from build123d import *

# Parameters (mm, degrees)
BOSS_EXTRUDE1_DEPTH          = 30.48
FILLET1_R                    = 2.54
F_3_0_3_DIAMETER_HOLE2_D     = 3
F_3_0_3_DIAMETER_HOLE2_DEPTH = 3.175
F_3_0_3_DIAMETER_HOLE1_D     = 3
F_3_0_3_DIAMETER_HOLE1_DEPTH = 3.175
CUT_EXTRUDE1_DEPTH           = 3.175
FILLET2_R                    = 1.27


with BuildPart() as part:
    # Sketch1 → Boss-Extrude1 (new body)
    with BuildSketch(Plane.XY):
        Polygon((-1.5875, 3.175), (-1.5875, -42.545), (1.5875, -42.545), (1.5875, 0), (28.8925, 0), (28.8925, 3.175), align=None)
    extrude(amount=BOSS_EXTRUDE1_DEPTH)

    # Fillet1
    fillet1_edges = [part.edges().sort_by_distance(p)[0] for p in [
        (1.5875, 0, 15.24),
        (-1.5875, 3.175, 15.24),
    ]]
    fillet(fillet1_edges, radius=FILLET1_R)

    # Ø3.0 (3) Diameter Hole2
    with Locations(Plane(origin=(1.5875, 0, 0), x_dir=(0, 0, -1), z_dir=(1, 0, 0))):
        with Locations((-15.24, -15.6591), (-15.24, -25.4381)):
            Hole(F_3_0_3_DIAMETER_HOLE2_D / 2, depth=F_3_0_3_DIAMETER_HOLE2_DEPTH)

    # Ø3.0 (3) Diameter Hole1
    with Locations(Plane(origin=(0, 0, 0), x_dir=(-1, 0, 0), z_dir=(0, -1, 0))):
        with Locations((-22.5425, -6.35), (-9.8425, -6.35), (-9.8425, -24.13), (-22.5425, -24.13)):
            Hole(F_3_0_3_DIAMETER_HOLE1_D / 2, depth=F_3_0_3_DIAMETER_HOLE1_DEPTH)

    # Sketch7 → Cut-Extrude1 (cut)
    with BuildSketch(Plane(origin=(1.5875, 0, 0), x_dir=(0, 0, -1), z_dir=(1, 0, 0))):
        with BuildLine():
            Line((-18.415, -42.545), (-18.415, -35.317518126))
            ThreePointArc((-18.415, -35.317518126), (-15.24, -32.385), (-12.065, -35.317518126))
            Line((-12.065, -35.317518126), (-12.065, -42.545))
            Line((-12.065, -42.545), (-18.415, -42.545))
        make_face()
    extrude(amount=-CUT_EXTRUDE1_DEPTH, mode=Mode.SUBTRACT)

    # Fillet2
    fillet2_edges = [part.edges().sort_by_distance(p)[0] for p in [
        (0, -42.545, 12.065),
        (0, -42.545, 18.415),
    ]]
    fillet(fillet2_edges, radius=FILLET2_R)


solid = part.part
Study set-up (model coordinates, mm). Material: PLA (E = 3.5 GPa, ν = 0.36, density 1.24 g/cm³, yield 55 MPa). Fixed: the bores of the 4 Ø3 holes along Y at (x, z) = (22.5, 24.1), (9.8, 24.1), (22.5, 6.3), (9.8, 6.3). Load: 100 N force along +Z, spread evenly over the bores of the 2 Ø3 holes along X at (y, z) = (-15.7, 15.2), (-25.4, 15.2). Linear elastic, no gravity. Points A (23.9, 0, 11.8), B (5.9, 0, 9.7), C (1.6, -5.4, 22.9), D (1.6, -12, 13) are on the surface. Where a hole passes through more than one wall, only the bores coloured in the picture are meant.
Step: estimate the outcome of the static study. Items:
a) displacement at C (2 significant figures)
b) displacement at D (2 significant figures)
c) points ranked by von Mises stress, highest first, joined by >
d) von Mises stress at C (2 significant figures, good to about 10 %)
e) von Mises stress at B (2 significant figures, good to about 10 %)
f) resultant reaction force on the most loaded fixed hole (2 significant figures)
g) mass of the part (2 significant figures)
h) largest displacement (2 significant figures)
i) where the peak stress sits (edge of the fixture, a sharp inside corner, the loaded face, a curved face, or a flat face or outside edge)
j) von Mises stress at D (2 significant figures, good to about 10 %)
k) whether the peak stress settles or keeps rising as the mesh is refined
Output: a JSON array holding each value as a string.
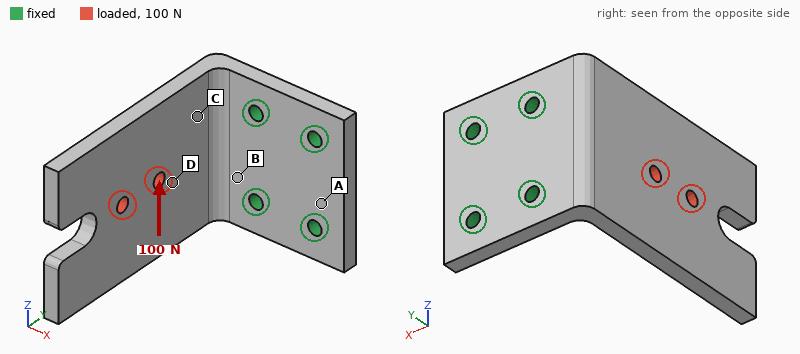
["0.14 mm", "0.20 mm", "B > C > D > A", "8.5 MPa", "12 MPa", "130 N", "8.4 g", "0.67 mm", "edge of the fixture", "4.3 MPa", "keeps rising"]
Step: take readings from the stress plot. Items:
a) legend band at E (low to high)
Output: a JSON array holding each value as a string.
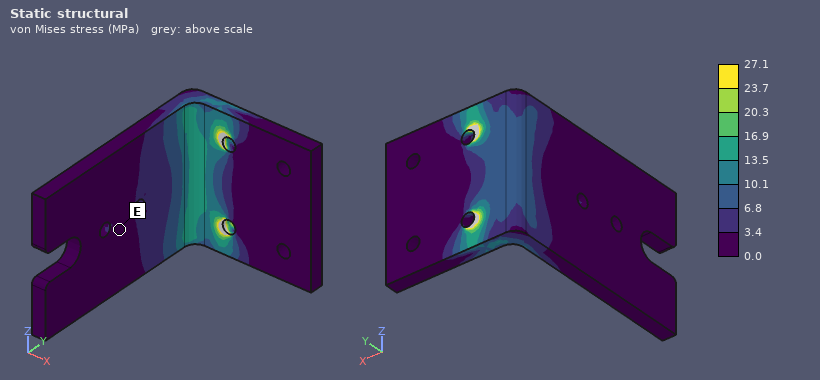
["0.0 to 3.4 MPa"]
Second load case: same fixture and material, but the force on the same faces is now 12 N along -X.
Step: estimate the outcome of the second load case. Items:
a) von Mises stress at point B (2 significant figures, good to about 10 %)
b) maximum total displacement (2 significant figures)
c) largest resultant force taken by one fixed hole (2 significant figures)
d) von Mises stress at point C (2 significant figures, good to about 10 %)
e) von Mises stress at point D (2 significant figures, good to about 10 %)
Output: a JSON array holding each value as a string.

["4.7 MPa", "0.63 mm", "6.3 N", "3.3 MPa", "1.9 MPa"]
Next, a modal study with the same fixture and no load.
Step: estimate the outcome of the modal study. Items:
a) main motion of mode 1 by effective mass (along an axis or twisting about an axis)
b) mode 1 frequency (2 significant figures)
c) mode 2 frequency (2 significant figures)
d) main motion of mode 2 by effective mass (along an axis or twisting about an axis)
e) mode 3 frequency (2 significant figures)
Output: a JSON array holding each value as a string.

["along X", "380 Hz", "1000 Hz", "along Z", "1400 Hz"]
